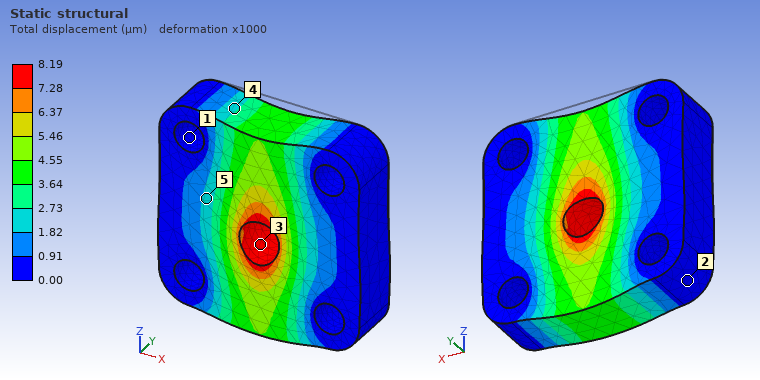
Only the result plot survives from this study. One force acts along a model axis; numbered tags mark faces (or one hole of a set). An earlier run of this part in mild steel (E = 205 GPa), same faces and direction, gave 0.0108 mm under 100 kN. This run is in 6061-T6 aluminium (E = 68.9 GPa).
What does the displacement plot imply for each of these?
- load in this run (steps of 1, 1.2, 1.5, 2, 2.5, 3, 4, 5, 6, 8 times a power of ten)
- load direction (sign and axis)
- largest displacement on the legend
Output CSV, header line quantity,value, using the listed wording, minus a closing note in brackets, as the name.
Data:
quantity,value
load in this run,25 kN
load direction,-Z
largest displacement on the legend,8.19 µm
